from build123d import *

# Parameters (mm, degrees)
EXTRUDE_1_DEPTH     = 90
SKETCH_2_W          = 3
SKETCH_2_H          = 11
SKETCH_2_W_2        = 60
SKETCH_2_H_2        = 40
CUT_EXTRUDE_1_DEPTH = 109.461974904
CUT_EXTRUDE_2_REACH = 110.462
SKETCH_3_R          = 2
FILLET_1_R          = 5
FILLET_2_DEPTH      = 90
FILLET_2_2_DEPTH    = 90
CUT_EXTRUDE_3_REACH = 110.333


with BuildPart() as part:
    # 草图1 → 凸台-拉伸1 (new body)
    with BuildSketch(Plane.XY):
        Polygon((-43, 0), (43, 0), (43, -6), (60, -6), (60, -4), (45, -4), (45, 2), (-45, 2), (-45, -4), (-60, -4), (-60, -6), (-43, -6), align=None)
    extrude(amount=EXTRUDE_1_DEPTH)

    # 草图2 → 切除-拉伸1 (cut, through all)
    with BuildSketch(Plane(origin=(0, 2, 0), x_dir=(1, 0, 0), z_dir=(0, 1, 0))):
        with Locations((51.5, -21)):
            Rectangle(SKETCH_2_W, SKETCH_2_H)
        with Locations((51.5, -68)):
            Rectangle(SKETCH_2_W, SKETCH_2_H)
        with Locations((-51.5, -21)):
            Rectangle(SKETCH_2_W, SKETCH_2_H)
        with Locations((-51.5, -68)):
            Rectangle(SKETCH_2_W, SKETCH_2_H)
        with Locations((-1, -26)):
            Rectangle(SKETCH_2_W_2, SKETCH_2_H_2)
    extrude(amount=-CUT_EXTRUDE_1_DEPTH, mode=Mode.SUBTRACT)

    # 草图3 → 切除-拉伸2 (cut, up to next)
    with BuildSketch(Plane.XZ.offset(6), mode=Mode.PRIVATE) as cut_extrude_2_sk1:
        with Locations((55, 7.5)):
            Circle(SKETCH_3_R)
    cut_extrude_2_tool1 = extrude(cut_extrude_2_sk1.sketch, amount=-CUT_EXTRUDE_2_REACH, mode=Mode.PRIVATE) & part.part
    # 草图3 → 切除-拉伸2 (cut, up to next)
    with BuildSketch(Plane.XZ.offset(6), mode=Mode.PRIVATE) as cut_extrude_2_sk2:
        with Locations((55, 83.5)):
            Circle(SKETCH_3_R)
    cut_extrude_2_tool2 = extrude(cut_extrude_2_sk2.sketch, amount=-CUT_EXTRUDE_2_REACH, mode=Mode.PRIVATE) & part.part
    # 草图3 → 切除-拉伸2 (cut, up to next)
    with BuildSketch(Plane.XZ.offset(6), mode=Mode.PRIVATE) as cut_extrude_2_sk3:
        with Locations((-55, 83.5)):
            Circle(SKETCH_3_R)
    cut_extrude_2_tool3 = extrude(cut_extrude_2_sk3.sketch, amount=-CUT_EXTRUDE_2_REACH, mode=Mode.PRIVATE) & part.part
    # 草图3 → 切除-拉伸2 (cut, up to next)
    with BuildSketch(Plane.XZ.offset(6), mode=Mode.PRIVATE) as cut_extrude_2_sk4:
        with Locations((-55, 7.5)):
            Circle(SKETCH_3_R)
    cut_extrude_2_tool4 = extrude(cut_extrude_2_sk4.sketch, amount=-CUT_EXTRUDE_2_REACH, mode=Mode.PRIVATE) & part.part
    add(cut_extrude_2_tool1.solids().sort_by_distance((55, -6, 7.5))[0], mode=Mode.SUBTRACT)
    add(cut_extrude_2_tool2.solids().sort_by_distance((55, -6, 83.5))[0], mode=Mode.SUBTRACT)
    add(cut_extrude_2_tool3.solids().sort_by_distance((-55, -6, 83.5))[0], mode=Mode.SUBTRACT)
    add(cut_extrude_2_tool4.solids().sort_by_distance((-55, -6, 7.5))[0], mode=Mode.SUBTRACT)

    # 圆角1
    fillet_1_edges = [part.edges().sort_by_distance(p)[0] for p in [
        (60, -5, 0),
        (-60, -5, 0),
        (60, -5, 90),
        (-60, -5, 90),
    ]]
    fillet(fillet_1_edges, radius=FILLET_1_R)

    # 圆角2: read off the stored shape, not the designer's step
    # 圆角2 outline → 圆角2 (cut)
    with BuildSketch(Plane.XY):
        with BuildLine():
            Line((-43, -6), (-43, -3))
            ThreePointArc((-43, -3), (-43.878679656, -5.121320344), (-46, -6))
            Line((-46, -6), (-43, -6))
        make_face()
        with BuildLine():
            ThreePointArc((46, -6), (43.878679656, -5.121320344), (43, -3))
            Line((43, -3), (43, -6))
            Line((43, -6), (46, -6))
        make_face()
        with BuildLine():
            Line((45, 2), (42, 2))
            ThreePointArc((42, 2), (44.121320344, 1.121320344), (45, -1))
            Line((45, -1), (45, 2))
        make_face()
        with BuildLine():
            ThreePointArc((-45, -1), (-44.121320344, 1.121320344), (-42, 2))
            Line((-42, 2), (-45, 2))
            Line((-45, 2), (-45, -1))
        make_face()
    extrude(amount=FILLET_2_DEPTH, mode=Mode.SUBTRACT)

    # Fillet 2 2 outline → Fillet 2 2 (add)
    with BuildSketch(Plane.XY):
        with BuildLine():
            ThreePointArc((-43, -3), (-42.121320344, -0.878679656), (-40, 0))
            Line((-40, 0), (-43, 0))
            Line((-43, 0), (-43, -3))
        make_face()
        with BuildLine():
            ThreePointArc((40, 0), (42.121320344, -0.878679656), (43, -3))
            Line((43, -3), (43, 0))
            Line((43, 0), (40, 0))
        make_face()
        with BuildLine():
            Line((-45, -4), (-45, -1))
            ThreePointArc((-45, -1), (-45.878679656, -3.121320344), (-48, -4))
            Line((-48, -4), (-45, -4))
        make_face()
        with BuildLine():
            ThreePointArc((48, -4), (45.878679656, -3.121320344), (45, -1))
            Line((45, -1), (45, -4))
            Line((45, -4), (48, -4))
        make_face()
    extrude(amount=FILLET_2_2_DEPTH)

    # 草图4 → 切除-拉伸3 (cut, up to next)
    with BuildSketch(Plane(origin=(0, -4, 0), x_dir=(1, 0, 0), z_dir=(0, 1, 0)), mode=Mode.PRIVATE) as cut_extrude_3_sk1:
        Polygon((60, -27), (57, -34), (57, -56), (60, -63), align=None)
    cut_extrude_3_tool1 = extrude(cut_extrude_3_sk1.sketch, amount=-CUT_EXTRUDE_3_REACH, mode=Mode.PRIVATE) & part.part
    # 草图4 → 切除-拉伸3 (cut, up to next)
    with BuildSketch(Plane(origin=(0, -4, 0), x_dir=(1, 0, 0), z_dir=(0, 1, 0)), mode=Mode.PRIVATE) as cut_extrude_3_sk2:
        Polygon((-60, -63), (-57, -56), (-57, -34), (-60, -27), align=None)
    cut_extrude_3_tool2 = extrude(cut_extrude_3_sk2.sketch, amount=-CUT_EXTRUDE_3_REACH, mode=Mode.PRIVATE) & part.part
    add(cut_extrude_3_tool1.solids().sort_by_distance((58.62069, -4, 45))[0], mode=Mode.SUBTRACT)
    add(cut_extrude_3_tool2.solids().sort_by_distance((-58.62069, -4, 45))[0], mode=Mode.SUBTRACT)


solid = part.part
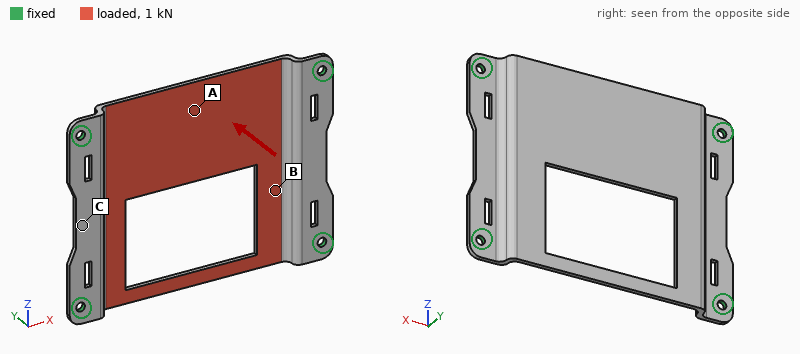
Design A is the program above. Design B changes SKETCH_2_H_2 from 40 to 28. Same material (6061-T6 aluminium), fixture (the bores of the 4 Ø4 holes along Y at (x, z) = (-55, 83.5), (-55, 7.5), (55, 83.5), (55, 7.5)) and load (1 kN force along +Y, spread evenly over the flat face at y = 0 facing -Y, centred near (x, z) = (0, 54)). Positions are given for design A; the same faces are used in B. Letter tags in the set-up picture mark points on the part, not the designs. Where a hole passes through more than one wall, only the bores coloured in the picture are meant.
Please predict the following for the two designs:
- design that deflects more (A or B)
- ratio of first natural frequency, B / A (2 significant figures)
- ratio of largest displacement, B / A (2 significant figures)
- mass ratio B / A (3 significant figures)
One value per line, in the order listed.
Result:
A
0.99
0.90
1.08
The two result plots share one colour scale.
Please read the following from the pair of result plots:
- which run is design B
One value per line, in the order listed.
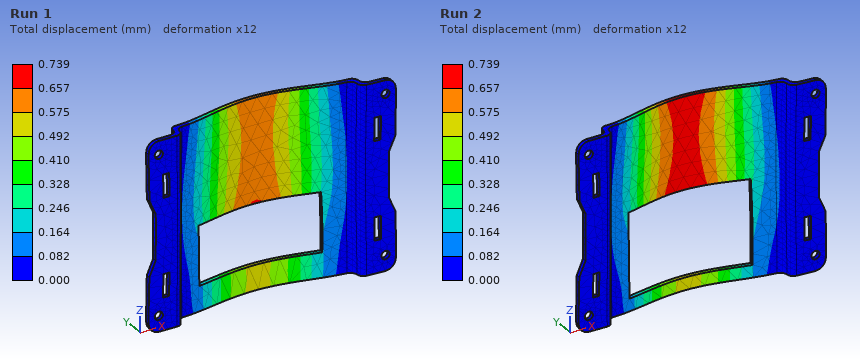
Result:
Run 1
